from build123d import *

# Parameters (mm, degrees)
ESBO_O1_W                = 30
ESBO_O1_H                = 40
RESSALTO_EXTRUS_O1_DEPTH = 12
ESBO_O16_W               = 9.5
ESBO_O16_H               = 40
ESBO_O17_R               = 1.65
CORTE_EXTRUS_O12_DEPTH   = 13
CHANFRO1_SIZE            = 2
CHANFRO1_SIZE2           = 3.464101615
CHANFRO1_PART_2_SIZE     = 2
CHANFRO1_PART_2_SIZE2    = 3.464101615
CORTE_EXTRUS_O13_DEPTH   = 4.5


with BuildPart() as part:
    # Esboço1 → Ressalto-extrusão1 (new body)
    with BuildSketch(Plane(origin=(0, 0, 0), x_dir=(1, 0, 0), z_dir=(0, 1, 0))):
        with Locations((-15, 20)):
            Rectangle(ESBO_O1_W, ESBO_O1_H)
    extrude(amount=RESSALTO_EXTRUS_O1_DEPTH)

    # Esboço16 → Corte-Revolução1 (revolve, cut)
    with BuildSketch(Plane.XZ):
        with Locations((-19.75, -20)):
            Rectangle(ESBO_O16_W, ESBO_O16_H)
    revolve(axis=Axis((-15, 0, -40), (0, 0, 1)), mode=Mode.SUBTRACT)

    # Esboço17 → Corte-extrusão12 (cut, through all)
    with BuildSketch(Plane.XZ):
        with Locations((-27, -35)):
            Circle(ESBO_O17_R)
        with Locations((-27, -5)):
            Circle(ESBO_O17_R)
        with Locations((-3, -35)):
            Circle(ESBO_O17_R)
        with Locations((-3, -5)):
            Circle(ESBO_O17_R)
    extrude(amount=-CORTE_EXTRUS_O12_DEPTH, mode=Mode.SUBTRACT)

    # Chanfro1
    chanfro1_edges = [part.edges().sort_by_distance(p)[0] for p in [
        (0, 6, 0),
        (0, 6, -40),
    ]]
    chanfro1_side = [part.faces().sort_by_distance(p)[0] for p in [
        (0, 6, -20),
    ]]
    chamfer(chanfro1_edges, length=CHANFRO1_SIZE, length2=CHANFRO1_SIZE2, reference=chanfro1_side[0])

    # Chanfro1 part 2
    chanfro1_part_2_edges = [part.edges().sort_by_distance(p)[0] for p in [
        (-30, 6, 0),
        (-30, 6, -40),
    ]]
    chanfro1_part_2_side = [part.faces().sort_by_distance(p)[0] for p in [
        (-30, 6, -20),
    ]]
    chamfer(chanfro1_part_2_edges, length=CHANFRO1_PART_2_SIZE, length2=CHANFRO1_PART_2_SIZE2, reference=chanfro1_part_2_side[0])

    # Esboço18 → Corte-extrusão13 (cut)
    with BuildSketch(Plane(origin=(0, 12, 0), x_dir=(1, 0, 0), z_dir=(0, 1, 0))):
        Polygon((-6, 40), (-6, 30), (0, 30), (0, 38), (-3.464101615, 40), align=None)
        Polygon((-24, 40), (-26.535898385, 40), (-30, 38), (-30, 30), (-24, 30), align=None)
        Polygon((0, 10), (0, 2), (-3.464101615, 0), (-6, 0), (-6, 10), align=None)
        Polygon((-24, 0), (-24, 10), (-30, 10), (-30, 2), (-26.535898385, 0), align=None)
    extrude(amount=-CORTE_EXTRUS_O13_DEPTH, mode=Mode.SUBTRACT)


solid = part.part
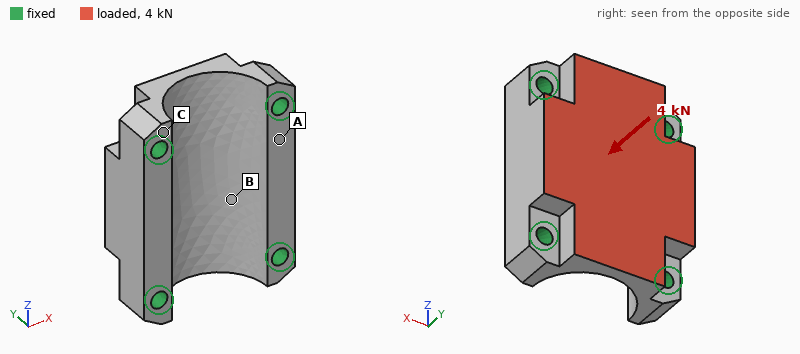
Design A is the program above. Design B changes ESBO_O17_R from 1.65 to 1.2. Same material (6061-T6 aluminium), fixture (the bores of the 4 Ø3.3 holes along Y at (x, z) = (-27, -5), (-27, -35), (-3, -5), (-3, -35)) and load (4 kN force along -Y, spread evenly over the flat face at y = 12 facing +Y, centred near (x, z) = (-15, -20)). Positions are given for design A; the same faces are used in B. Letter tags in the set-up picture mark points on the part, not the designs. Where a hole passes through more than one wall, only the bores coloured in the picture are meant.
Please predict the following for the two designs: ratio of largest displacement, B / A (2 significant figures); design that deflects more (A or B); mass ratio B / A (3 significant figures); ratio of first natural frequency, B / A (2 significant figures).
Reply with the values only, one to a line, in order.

1.1
B
1.02
0.94
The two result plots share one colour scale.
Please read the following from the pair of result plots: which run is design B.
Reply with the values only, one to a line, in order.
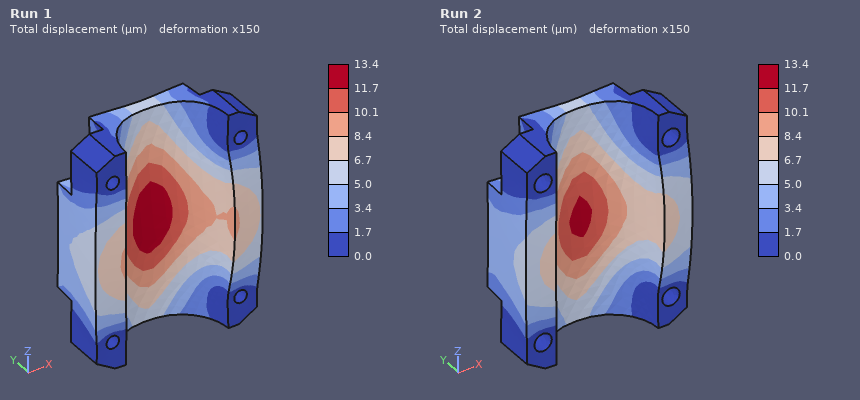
Run 1
